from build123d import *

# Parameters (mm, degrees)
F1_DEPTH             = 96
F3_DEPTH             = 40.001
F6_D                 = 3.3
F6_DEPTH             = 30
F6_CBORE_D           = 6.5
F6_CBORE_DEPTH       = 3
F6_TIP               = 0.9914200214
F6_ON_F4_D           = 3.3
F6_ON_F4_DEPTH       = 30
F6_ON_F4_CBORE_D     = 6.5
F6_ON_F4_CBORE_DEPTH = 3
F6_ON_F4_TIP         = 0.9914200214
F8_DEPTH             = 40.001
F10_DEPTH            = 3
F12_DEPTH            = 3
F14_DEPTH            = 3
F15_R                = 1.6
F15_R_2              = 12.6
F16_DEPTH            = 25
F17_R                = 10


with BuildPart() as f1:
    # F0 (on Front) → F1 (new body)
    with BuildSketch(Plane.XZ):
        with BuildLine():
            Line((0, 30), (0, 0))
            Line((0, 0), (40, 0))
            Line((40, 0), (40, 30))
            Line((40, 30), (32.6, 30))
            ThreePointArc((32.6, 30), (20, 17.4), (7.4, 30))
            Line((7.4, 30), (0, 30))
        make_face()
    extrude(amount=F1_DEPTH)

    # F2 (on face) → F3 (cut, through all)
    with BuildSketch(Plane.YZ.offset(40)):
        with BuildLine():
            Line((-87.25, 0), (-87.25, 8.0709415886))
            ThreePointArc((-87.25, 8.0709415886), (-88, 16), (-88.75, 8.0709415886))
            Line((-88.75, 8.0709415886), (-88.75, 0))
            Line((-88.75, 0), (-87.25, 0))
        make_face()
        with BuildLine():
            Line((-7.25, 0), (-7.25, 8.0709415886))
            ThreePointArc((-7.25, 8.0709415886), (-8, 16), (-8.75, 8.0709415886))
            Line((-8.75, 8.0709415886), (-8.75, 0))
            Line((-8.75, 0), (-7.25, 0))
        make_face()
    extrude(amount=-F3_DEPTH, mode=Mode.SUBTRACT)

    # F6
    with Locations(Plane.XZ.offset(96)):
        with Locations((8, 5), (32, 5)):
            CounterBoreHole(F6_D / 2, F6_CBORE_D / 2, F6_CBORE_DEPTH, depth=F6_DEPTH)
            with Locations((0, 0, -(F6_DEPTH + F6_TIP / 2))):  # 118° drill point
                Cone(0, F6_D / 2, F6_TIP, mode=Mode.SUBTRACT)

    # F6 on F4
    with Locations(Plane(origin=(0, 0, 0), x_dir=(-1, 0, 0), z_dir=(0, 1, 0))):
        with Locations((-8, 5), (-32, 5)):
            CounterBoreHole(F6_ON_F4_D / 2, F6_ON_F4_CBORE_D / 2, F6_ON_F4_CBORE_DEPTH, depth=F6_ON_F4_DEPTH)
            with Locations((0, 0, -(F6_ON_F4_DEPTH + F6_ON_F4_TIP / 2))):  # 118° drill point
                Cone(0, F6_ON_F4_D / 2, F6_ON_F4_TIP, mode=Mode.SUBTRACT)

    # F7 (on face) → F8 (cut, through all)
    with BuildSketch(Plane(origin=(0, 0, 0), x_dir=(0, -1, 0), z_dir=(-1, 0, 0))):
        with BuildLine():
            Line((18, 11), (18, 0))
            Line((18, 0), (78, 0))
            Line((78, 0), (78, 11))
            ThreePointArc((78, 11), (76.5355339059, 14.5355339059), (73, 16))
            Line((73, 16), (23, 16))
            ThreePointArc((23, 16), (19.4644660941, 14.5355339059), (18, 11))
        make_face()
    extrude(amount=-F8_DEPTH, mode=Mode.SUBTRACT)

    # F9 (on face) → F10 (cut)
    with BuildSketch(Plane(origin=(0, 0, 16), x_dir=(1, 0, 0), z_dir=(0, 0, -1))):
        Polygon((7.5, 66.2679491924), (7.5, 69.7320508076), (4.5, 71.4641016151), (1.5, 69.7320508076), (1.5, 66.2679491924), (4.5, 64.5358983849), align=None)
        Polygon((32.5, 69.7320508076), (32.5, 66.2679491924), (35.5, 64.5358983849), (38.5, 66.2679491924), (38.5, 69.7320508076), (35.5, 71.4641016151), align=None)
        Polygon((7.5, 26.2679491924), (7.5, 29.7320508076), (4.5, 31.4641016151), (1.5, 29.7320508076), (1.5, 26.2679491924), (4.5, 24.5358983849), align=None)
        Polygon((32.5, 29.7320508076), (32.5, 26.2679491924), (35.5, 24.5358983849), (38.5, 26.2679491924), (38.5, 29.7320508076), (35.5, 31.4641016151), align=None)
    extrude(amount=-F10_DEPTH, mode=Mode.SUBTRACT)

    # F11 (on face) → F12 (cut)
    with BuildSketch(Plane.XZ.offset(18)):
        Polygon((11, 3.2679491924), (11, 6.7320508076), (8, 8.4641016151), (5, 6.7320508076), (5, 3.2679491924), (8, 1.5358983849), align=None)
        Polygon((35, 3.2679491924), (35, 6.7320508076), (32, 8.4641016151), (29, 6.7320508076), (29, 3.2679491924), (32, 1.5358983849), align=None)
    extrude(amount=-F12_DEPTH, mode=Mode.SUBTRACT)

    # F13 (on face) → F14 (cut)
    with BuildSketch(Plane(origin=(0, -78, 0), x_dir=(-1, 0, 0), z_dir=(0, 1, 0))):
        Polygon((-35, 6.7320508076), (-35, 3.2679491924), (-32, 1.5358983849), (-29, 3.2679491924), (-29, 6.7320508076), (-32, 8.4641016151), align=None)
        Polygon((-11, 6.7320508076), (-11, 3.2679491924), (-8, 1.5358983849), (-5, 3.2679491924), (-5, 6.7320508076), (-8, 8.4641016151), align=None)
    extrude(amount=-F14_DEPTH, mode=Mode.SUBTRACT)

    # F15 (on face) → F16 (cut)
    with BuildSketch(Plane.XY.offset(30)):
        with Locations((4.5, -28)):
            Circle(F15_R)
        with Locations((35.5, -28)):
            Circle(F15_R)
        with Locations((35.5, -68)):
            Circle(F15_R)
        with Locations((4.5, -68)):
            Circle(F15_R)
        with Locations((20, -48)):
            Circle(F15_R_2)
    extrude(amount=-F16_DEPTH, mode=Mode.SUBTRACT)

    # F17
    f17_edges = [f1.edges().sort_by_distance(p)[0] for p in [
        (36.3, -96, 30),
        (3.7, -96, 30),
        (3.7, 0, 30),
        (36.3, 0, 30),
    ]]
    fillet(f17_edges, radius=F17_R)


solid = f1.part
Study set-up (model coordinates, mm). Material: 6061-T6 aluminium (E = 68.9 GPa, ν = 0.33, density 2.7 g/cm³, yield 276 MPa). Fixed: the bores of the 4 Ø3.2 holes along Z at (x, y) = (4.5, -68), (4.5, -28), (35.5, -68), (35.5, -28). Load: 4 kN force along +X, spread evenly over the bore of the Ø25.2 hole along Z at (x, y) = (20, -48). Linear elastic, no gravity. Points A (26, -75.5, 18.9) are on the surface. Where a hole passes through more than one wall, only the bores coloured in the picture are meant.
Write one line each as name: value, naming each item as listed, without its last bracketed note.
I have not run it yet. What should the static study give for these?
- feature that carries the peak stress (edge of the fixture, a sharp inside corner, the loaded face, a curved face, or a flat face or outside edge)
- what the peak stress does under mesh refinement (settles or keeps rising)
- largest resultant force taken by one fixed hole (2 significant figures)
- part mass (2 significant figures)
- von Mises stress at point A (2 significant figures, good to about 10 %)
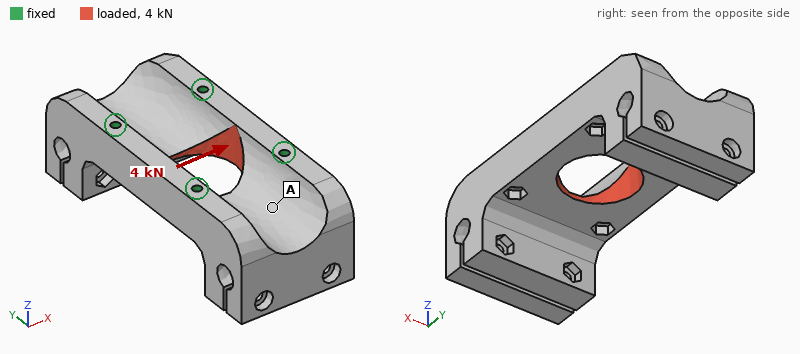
feature that carries the peak stress: edge of the fixture
what the peak stress does under mesh refinement: keeps rising
largest resultant force taken by one fixed hole: 1.0 kN
part mass: 120 g
von Mises stress at point A: 9.4 MPa
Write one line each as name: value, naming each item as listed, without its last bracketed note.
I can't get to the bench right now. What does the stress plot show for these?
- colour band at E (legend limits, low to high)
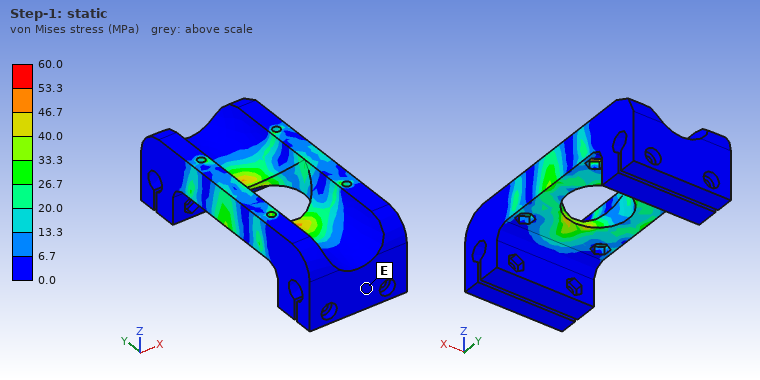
colour band at E: 0.0 to 6.7 MPa
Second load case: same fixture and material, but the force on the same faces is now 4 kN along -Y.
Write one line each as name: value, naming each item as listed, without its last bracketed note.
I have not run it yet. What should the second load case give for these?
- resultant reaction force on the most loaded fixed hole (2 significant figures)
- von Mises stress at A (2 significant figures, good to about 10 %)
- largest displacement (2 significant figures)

resultant reaction force on the most loaded fixed hole: 1.0 kN
von Mises stress at A: 2.1 MPa
largest displacement: 3.7 µm
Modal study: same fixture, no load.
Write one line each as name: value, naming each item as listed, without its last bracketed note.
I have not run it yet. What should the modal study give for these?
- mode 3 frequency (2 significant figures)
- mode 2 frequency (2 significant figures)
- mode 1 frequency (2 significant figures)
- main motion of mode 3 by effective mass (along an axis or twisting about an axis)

mode 3 frequency: 8400 Hz
mode 2 frequency: 5300 Hz
mode 1 frequency: 5200 Hz
main motion of mode 3 by effective mass: twisting about Y
